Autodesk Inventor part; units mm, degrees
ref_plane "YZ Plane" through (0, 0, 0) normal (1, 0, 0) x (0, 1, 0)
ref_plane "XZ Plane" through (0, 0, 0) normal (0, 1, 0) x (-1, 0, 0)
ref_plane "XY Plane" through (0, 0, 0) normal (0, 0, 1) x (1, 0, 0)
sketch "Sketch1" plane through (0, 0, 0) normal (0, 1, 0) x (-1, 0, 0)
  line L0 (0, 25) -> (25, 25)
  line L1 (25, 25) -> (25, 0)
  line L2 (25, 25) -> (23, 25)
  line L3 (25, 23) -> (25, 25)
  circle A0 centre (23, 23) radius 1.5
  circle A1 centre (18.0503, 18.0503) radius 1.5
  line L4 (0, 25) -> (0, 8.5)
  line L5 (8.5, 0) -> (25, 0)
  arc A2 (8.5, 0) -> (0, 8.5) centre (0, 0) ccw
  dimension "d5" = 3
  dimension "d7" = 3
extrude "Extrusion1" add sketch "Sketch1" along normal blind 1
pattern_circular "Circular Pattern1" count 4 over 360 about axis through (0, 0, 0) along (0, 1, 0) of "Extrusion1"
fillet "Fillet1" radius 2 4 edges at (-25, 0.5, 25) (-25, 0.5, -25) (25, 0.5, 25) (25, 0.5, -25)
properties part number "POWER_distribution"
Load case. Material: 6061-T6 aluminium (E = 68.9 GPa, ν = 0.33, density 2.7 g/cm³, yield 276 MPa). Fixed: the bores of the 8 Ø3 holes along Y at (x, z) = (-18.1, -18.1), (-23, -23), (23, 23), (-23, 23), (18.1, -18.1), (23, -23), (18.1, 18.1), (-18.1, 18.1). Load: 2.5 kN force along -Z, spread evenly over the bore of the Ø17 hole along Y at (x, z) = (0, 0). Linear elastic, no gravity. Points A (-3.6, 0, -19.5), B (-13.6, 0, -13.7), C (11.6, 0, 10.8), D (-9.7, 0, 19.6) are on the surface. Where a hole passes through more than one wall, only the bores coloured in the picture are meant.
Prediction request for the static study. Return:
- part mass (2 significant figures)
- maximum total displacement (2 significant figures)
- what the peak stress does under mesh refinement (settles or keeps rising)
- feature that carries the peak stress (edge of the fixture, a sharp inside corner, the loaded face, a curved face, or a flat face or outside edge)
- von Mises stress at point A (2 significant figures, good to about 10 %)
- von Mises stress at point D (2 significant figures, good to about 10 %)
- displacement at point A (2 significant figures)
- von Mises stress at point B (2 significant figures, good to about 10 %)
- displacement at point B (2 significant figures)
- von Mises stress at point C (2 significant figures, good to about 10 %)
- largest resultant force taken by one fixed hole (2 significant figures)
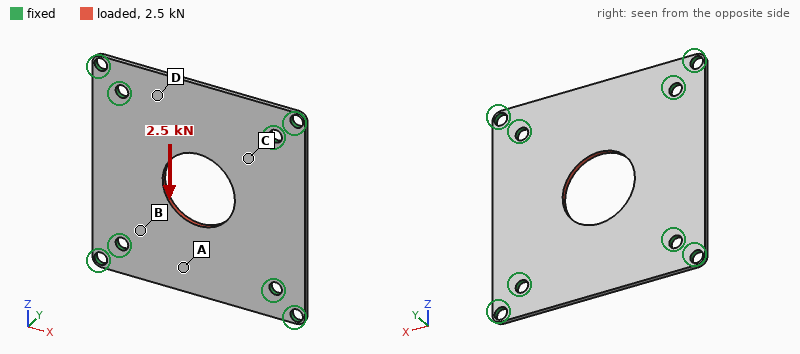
6.0 g
21 µm
keeps rising
edge of the fixture
21 MPa
34 MPa
16 µm
59 MPa
7.0 µm
50 MPa
570 N
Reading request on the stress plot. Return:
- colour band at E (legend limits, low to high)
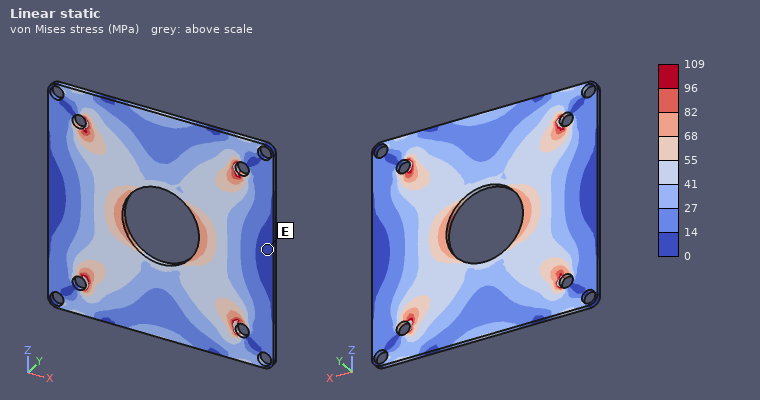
0 to 14 MPa
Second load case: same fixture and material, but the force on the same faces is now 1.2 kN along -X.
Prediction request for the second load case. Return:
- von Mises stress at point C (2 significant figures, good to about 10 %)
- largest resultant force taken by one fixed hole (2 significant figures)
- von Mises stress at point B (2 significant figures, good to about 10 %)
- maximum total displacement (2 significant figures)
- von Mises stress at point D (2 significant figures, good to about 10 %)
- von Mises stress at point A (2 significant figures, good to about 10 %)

24 MPa
270 N
29 MPa
10 µm
14 MPa
9.9 MPa
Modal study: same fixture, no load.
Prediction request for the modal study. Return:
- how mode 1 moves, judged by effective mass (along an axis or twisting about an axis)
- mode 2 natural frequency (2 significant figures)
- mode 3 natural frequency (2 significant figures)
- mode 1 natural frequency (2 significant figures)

along Y
4500 Hz
4500 Hz
3400 Hz
